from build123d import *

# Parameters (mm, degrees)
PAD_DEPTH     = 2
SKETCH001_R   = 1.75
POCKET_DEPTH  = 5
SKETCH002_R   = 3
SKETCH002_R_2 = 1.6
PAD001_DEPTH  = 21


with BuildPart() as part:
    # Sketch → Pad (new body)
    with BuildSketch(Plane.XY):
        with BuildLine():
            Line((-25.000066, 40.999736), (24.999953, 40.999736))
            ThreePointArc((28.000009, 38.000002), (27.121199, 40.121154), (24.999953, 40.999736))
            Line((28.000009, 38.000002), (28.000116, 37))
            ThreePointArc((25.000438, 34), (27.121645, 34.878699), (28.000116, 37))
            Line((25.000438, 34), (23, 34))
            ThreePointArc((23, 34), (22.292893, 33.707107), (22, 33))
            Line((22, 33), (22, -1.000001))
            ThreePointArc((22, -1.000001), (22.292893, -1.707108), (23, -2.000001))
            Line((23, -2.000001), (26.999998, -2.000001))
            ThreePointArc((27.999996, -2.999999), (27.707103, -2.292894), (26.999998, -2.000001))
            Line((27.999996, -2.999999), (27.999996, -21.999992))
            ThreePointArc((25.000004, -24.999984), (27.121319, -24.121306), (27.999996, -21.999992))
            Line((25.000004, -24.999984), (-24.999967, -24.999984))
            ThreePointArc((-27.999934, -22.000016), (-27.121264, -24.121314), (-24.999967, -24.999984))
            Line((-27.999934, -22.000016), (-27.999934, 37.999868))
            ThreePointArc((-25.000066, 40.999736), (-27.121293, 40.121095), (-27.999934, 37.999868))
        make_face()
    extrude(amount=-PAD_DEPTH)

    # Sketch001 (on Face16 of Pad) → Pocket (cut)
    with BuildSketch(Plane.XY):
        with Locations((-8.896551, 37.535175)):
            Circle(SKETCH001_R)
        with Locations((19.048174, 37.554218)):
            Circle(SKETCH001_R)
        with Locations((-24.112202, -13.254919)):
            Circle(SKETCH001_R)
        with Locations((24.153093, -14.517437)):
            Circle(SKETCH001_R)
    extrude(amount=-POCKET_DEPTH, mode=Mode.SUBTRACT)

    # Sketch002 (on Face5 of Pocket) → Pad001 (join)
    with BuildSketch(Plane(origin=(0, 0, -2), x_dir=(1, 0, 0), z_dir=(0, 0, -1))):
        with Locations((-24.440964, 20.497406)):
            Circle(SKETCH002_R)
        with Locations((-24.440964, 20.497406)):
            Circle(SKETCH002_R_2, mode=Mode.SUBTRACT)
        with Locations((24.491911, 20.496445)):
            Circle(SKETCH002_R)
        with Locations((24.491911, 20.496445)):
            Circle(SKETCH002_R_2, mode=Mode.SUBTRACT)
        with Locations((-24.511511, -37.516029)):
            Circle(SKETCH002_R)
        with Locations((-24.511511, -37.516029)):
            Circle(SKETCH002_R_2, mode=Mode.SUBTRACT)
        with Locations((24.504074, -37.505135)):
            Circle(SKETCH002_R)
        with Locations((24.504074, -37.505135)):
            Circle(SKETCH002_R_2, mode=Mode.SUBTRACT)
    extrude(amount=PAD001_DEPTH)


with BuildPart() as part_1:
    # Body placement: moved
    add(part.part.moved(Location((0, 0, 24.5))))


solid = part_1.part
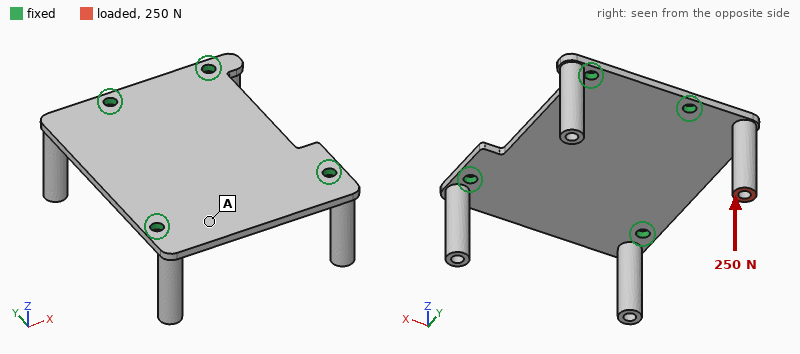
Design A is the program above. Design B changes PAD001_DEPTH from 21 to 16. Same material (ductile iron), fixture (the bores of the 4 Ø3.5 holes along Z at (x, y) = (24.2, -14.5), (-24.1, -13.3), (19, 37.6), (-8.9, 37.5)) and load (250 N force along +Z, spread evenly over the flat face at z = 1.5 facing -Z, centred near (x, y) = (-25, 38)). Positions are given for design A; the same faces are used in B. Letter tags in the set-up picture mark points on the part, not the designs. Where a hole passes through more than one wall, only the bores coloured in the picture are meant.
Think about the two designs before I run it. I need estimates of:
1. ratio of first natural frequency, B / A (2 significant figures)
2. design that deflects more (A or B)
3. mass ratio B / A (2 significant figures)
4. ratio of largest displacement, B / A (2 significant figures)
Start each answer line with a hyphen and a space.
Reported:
- 1.2
- A
- 0.95
- 0.84
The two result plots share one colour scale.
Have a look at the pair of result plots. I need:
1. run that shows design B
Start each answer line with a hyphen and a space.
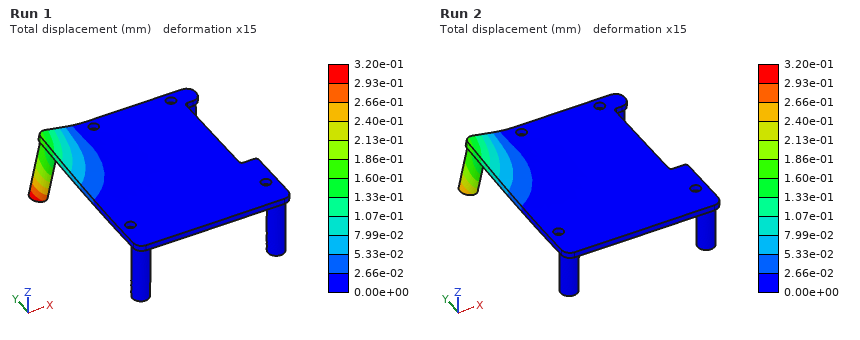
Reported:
- Run 2
